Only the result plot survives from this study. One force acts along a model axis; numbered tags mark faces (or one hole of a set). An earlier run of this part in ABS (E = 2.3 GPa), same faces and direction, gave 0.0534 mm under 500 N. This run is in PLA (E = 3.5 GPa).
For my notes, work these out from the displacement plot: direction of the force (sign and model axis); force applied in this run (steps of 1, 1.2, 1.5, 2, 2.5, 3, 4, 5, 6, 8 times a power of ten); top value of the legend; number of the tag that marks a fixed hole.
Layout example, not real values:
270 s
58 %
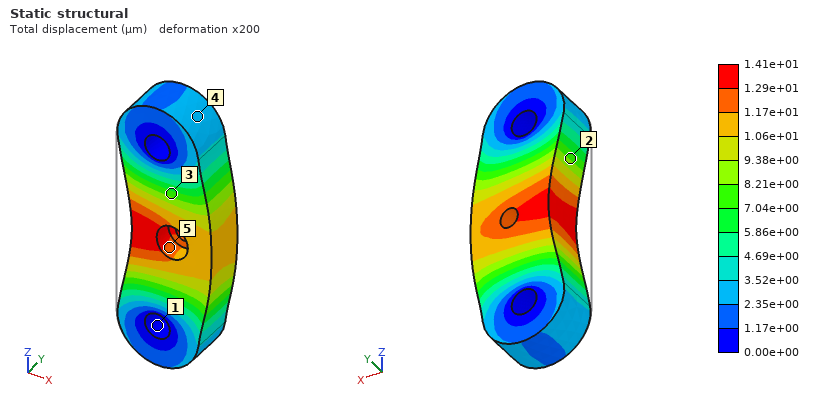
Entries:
+X
200 N
1.41e+01 µm
1
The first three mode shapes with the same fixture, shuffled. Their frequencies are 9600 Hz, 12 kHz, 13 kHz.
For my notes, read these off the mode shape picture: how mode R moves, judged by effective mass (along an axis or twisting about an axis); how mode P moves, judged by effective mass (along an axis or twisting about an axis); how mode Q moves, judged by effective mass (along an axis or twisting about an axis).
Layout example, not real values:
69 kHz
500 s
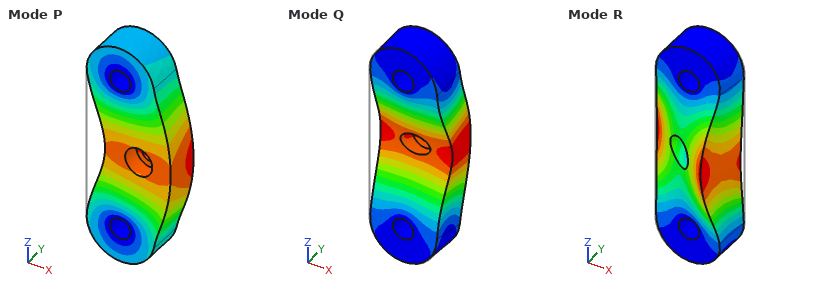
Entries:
twisting about Z
along X
along Y
